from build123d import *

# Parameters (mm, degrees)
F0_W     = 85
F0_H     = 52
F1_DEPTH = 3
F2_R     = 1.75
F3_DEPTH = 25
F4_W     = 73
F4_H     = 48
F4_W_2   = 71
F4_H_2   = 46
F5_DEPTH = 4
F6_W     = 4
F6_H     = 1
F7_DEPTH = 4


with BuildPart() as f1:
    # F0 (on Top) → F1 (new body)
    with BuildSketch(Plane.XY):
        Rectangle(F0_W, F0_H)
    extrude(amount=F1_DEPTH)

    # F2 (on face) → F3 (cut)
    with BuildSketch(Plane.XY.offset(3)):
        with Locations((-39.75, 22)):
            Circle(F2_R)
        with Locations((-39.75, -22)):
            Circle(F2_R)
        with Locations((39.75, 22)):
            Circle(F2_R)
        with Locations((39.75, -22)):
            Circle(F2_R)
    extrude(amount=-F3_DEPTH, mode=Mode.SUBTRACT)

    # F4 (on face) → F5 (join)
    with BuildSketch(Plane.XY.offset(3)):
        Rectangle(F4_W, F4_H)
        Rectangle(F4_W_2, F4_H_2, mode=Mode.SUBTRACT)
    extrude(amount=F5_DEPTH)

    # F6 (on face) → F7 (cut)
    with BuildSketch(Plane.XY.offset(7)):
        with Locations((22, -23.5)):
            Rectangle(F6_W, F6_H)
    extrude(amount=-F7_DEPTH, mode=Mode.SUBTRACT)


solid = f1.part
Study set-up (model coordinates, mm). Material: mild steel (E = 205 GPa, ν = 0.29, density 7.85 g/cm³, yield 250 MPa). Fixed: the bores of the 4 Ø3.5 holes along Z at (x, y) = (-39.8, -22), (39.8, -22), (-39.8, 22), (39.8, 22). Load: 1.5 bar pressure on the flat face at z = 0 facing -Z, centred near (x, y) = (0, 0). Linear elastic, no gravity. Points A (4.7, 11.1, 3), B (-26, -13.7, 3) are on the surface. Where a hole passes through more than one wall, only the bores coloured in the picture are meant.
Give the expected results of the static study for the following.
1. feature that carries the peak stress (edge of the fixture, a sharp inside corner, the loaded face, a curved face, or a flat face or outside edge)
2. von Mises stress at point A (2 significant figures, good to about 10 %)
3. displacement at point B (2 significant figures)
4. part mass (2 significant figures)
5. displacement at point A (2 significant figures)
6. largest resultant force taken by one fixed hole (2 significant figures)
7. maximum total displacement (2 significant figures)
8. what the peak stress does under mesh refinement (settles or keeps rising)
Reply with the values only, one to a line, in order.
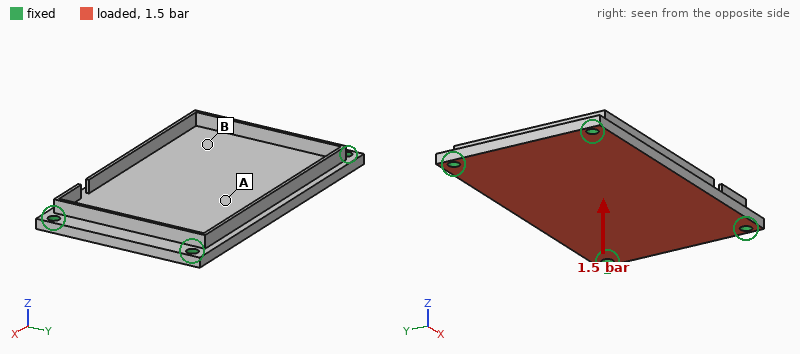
edge of the fixture
18 MPa
15 µm
110 g
33 µm
170 N
35 µm
keeps rising
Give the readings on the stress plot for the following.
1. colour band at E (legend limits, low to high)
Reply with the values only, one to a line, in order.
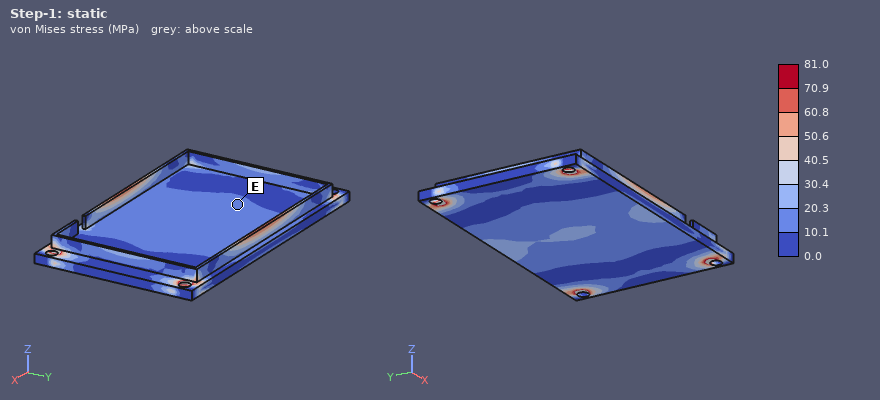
10.1 to 20.3 MPa
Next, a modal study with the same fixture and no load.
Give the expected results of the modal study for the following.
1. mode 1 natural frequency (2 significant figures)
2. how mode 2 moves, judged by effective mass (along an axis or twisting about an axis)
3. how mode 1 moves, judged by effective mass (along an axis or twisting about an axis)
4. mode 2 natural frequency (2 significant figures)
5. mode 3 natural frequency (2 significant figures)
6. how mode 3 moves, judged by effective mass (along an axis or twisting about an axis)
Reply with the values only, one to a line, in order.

2400 Hz
twisting about X
along Z
3900 Hz
6300 Hz
twisting about Y
